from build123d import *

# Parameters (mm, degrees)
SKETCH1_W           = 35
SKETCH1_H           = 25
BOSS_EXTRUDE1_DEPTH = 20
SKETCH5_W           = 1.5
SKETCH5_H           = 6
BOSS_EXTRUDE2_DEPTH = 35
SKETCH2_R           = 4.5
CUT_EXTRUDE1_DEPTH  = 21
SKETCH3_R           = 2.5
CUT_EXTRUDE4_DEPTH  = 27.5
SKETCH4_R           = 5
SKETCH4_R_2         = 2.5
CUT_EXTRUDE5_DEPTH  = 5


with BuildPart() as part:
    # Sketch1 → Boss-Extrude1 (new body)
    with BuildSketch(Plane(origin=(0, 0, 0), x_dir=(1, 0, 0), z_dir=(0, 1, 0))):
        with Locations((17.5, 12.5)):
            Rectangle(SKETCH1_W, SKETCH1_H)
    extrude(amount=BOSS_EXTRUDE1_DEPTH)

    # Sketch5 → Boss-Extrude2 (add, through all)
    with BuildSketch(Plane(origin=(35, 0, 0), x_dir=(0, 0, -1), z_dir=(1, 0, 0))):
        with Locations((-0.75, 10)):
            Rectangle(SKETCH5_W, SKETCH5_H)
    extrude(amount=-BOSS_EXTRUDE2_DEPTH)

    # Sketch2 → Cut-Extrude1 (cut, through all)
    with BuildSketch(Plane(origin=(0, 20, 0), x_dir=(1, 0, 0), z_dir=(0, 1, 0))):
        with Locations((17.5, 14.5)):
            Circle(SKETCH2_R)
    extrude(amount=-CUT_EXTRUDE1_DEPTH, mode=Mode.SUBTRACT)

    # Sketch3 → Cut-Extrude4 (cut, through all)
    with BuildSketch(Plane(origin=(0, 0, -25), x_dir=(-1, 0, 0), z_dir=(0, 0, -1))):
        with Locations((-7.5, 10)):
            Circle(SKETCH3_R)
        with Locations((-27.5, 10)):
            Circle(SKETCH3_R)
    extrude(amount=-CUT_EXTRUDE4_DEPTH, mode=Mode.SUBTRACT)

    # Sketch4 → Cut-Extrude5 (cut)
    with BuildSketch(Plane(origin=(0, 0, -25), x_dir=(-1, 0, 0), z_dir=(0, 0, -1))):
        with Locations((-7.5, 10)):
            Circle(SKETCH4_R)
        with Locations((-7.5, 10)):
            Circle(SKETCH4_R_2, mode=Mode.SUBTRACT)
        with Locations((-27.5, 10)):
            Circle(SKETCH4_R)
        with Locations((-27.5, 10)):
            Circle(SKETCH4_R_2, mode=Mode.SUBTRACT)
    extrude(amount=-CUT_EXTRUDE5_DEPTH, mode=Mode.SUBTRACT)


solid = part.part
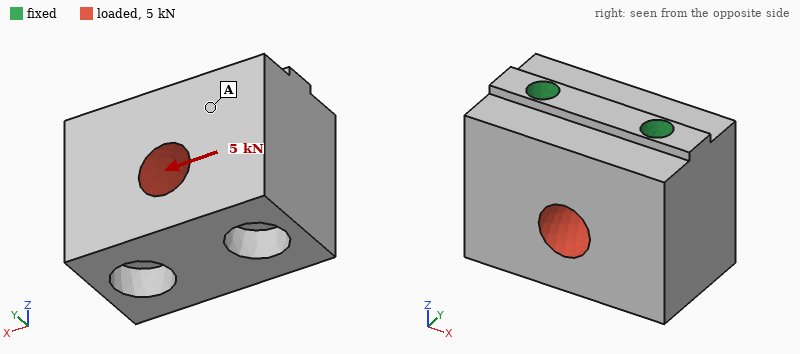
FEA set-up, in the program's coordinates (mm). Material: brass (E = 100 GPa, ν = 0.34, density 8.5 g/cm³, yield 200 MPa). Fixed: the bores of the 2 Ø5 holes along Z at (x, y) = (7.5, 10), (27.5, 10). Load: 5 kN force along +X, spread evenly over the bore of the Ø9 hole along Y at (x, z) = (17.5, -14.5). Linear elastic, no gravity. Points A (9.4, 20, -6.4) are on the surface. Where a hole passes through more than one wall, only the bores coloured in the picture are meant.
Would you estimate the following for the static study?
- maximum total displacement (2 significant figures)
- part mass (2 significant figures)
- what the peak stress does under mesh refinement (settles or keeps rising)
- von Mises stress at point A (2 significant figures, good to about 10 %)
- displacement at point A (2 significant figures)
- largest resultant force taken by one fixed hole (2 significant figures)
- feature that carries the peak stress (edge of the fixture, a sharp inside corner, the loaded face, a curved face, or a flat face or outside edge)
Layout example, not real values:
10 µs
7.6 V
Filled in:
1.5 µm
130 g
keeps rising
3.7 MPa
0.46 µm
2.5 kN
edge of the fixture
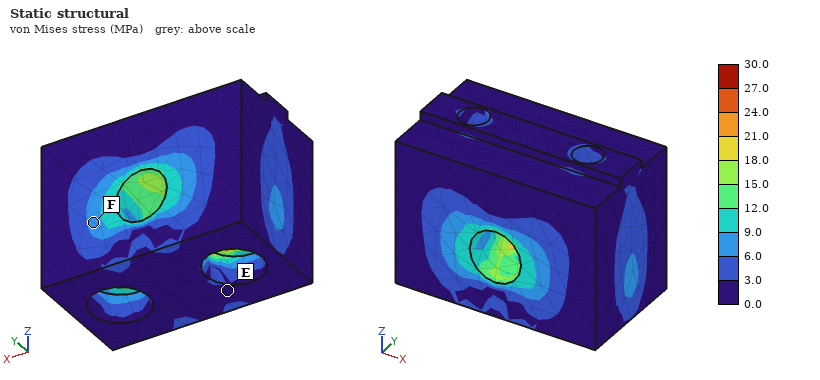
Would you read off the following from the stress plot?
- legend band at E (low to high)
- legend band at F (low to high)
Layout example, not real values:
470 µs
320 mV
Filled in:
0.0 to 3.0 MPa
6.0 to 9.0 MPa
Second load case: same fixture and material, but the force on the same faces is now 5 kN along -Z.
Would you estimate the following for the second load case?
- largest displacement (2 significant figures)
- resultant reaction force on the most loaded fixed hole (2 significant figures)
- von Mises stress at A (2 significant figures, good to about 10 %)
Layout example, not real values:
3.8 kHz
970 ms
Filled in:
2.4 µm
2.5 kN
5.9 MPa
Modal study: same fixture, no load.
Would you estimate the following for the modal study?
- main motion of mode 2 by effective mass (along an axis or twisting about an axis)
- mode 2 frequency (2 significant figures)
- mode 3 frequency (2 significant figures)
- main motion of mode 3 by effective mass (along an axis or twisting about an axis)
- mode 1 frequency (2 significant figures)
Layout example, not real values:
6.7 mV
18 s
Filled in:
twisting about Z
33 kHz
35 kHz
along X
28 kHz
